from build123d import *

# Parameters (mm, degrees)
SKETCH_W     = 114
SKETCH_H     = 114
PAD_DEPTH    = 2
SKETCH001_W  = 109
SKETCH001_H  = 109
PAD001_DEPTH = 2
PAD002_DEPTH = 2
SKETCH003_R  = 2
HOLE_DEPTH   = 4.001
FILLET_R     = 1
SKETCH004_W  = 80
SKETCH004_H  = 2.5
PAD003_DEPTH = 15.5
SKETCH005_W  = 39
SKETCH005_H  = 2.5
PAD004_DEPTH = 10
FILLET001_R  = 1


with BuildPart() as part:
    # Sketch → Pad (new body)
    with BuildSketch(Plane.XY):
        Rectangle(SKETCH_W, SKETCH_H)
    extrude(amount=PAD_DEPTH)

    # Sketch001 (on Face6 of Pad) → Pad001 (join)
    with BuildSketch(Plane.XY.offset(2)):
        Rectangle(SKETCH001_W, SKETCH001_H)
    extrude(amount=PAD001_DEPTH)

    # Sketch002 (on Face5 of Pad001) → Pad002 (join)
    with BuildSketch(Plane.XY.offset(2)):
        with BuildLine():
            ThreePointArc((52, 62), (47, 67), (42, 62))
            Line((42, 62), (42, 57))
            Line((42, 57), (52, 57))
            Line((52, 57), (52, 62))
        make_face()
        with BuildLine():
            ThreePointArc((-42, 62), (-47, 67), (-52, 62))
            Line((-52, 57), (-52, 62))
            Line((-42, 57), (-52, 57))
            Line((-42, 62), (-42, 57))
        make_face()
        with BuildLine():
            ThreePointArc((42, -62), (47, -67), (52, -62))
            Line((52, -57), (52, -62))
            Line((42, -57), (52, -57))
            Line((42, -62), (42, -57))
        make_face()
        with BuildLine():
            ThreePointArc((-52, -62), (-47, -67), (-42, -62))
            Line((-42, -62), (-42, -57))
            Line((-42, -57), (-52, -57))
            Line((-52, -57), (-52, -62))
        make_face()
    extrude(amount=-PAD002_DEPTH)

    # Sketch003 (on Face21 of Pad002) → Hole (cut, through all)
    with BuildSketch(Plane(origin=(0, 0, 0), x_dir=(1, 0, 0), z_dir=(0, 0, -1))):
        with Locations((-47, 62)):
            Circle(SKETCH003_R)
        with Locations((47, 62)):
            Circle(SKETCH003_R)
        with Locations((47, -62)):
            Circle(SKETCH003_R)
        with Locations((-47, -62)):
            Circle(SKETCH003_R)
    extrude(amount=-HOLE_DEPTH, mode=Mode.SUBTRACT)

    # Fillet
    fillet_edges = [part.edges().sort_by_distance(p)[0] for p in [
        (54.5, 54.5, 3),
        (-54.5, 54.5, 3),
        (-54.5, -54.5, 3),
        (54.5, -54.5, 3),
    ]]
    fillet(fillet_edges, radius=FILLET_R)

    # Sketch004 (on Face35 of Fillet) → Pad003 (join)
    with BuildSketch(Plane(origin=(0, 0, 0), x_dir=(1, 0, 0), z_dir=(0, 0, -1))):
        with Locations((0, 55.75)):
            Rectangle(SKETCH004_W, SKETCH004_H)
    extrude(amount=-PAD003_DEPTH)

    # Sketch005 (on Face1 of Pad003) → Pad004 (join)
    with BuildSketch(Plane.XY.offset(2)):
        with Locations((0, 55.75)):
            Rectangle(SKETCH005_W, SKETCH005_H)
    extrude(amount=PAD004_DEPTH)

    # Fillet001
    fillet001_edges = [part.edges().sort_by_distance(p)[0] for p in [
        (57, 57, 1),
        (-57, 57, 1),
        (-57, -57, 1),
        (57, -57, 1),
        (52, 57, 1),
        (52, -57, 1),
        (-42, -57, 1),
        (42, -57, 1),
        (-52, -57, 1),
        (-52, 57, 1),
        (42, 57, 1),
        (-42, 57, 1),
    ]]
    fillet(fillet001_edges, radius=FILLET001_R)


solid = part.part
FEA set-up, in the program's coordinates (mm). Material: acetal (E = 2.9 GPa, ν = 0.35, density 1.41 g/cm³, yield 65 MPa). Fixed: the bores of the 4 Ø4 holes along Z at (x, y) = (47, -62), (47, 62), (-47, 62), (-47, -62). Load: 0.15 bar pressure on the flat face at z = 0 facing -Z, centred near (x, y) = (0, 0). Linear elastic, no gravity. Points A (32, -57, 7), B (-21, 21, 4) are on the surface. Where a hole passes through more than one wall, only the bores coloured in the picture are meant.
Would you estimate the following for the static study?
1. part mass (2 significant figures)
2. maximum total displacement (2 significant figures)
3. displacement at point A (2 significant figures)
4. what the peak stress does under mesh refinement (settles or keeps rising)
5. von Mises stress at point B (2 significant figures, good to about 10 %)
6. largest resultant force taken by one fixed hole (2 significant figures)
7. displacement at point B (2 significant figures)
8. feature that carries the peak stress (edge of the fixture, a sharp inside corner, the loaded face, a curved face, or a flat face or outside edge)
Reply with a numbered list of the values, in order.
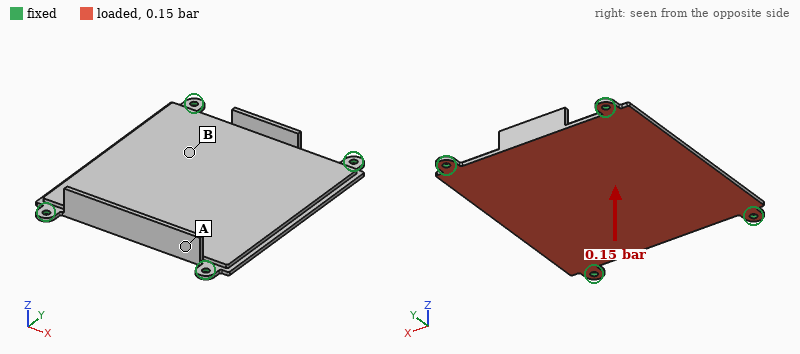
1. 76 g
2. 1.9 mm
3. 0.30 mm
4. keeps rising
5. 5.9 MPa
6. 160 N
7. 1.6 mm
8. edge of the fixture
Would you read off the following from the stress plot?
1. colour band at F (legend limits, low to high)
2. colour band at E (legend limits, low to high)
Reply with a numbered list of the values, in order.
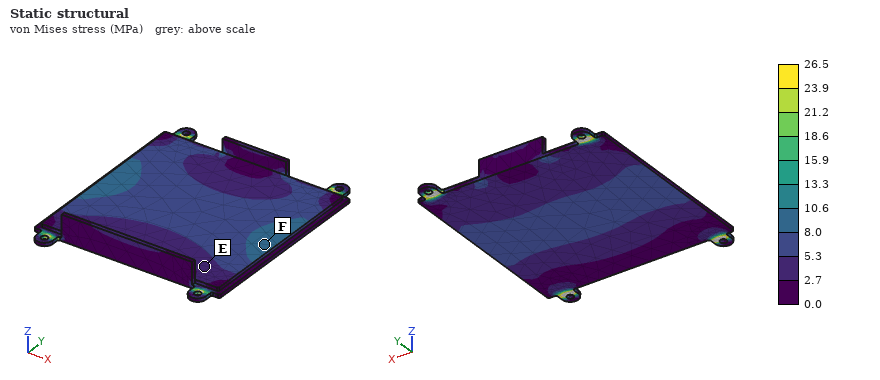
1. 8.0 to 10.6 MPa
2. 2.7 to 5.3 MPa
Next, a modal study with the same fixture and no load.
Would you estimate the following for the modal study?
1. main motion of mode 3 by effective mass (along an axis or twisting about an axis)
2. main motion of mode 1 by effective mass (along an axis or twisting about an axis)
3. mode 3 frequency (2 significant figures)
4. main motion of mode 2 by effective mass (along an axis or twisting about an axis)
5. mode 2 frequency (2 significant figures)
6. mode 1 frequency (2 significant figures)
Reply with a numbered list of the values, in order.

1. twisting about X
2. along Z
3. 500 Hz
4. twisting about Y
5. 350 Hz
6. 220 Hz
